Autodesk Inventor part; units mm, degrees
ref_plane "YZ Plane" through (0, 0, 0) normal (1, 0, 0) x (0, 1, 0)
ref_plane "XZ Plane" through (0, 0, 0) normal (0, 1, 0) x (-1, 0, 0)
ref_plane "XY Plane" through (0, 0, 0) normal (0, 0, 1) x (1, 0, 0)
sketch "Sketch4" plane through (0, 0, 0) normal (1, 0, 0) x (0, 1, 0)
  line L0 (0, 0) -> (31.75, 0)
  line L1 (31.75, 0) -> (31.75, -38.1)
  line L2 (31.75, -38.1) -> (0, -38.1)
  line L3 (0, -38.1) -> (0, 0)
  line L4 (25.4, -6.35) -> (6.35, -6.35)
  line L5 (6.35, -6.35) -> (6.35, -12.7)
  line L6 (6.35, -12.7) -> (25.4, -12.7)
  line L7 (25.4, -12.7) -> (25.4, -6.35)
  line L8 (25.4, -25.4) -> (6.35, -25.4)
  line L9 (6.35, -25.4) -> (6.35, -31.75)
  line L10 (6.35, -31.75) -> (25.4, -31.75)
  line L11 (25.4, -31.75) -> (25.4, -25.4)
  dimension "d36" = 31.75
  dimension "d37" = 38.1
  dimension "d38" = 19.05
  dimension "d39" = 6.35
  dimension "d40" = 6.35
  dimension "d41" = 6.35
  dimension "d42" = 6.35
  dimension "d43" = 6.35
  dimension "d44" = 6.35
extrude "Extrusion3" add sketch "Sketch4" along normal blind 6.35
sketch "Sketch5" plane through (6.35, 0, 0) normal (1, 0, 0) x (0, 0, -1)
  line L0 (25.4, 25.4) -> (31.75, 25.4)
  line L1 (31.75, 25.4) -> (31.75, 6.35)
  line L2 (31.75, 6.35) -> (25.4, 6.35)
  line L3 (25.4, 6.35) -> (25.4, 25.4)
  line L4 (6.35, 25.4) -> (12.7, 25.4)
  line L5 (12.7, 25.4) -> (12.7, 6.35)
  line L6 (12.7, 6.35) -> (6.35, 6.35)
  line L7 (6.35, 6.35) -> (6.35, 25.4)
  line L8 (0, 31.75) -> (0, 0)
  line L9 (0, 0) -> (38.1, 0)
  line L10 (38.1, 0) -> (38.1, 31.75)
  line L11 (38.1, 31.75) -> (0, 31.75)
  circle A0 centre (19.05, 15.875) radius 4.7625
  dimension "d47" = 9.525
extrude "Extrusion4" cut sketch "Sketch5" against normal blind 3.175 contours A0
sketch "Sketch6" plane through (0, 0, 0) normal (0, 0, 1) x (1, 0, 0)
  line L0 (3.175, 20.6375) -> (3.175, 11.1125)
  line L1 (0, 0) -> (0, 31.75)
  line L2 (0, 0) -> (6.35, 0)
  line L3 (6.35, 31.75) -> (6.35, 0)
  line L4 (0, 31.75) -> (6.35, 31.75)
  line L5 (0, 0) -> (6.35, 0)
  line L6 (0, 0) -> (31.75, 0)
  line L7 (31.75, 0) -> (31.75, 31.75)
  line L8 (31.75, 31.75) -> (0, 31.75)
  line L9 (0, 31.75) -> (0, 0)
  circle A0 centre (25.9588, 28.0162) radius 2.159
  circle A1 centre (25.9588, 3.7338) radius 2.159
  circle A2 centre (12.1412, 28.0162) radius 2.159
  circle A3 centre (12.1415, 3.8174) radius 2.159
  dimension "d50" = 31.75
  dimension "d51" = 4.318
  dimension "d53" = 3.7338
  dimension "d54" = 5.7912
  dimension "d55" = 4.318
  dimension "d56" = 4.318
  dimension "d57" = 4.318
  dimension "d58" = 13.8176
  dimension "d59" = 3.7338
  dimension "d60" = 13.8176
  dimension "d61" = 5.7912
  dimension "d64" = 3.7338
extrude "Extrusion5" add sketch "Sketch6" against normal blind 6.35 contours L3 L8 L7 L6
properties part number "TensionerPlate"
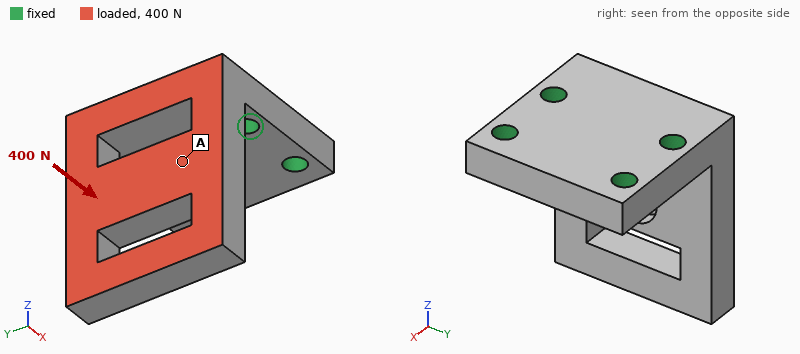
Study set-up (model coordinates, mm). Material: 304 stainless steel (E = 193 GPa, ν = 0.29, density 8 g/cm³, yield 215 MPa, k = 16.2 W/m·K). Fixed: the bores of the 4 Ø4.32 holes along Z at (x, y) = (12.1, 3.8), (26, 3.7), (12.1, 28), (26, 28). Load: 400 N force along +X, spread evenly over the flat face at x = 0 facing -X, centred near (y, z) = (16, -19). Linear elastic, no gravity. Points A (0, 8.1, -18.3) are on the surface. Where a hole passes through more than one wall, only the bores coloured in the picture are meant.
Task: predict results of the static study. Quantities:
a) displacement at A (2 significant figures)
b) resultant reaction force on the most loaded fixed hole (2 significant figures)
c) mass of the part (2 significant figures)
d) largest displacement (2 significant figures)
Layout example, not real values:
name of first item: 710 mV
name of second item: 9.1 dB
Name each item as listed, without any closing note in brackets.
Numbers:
displacement at A: 18 µm
resultant reaction force on the most loaded fixed hole: 190 N
mass of the part: 85 g
largest displacement: 49 µm
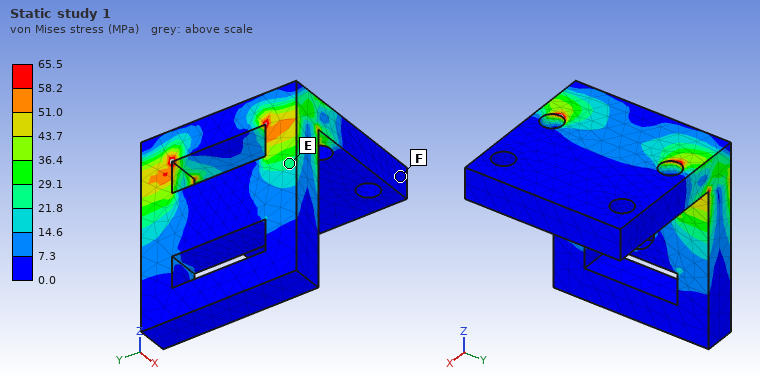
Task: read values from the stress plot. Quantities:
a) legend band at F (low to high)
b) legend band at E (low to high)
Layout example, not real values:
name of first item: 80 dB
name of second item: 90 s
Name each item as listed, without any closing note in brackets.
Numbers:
legend band at F: 0.0 to 7.3 MPa
legend band at E: 21.8 to 29.1 MPa
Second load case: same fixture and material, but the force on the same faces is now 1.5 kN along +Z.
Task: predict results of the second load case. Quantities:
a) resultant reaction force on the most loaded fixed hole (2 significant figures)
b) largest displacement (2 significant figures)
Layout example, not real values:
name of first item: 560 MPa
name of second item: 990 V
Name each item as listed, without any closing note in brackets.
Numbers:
resultant reaction force on the most loaded fixed hole: 870 N
largest displacement: 62 µm
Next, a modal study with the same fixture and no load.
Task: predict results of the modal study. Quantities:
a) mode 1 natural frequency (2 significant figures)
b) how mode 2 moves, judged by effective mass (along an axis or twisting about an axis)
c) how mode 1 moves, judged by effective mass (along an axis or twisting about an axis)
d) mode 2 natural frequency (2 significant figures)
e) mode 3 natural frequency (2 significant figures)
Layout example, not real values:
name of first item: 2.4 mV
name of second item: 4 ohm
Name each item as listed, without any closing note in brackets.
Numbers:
mode 1 natural frequency: 2500 Hz
how mode 2 moves, judged by effective mass: along Y
how mode 1 moves, judged by effective mass: along X
mode 2 natural frequency: 6000 Hz
mode 3 natural frequency: 8000 Hz
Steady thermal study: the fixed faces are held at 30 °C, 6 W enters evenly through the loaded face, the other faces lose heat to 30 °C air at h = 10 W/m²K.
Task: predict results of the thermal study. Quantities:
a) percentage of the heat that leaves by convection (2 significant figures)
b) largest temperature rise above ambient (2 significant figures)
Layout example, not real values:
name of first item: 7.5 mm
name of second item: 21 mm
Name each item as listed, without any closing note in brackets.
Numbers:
percentage of the heat that leaves by convection: 18 %
largest temperature rise above ambient: 62 K
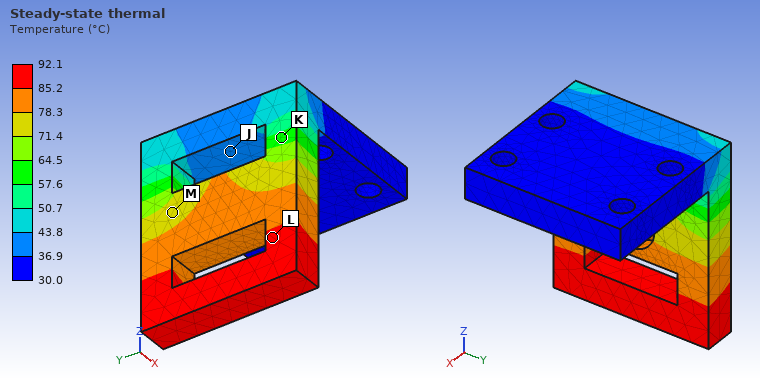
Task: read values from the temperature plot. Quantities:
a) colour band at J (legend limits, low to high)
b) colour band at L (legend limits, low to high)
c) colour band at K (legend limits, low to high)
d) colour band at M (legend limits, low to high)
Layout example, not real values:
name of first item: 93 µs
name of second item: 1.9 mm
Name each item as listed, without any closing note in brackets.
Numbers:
colour band at J: 36.9 to 43.8 °C
colour band at L: 85.2 to 92.1 °C
colour band at K: 57.6 to 64.5 °C
colour band at M: 71.4 to 78.3 °C
